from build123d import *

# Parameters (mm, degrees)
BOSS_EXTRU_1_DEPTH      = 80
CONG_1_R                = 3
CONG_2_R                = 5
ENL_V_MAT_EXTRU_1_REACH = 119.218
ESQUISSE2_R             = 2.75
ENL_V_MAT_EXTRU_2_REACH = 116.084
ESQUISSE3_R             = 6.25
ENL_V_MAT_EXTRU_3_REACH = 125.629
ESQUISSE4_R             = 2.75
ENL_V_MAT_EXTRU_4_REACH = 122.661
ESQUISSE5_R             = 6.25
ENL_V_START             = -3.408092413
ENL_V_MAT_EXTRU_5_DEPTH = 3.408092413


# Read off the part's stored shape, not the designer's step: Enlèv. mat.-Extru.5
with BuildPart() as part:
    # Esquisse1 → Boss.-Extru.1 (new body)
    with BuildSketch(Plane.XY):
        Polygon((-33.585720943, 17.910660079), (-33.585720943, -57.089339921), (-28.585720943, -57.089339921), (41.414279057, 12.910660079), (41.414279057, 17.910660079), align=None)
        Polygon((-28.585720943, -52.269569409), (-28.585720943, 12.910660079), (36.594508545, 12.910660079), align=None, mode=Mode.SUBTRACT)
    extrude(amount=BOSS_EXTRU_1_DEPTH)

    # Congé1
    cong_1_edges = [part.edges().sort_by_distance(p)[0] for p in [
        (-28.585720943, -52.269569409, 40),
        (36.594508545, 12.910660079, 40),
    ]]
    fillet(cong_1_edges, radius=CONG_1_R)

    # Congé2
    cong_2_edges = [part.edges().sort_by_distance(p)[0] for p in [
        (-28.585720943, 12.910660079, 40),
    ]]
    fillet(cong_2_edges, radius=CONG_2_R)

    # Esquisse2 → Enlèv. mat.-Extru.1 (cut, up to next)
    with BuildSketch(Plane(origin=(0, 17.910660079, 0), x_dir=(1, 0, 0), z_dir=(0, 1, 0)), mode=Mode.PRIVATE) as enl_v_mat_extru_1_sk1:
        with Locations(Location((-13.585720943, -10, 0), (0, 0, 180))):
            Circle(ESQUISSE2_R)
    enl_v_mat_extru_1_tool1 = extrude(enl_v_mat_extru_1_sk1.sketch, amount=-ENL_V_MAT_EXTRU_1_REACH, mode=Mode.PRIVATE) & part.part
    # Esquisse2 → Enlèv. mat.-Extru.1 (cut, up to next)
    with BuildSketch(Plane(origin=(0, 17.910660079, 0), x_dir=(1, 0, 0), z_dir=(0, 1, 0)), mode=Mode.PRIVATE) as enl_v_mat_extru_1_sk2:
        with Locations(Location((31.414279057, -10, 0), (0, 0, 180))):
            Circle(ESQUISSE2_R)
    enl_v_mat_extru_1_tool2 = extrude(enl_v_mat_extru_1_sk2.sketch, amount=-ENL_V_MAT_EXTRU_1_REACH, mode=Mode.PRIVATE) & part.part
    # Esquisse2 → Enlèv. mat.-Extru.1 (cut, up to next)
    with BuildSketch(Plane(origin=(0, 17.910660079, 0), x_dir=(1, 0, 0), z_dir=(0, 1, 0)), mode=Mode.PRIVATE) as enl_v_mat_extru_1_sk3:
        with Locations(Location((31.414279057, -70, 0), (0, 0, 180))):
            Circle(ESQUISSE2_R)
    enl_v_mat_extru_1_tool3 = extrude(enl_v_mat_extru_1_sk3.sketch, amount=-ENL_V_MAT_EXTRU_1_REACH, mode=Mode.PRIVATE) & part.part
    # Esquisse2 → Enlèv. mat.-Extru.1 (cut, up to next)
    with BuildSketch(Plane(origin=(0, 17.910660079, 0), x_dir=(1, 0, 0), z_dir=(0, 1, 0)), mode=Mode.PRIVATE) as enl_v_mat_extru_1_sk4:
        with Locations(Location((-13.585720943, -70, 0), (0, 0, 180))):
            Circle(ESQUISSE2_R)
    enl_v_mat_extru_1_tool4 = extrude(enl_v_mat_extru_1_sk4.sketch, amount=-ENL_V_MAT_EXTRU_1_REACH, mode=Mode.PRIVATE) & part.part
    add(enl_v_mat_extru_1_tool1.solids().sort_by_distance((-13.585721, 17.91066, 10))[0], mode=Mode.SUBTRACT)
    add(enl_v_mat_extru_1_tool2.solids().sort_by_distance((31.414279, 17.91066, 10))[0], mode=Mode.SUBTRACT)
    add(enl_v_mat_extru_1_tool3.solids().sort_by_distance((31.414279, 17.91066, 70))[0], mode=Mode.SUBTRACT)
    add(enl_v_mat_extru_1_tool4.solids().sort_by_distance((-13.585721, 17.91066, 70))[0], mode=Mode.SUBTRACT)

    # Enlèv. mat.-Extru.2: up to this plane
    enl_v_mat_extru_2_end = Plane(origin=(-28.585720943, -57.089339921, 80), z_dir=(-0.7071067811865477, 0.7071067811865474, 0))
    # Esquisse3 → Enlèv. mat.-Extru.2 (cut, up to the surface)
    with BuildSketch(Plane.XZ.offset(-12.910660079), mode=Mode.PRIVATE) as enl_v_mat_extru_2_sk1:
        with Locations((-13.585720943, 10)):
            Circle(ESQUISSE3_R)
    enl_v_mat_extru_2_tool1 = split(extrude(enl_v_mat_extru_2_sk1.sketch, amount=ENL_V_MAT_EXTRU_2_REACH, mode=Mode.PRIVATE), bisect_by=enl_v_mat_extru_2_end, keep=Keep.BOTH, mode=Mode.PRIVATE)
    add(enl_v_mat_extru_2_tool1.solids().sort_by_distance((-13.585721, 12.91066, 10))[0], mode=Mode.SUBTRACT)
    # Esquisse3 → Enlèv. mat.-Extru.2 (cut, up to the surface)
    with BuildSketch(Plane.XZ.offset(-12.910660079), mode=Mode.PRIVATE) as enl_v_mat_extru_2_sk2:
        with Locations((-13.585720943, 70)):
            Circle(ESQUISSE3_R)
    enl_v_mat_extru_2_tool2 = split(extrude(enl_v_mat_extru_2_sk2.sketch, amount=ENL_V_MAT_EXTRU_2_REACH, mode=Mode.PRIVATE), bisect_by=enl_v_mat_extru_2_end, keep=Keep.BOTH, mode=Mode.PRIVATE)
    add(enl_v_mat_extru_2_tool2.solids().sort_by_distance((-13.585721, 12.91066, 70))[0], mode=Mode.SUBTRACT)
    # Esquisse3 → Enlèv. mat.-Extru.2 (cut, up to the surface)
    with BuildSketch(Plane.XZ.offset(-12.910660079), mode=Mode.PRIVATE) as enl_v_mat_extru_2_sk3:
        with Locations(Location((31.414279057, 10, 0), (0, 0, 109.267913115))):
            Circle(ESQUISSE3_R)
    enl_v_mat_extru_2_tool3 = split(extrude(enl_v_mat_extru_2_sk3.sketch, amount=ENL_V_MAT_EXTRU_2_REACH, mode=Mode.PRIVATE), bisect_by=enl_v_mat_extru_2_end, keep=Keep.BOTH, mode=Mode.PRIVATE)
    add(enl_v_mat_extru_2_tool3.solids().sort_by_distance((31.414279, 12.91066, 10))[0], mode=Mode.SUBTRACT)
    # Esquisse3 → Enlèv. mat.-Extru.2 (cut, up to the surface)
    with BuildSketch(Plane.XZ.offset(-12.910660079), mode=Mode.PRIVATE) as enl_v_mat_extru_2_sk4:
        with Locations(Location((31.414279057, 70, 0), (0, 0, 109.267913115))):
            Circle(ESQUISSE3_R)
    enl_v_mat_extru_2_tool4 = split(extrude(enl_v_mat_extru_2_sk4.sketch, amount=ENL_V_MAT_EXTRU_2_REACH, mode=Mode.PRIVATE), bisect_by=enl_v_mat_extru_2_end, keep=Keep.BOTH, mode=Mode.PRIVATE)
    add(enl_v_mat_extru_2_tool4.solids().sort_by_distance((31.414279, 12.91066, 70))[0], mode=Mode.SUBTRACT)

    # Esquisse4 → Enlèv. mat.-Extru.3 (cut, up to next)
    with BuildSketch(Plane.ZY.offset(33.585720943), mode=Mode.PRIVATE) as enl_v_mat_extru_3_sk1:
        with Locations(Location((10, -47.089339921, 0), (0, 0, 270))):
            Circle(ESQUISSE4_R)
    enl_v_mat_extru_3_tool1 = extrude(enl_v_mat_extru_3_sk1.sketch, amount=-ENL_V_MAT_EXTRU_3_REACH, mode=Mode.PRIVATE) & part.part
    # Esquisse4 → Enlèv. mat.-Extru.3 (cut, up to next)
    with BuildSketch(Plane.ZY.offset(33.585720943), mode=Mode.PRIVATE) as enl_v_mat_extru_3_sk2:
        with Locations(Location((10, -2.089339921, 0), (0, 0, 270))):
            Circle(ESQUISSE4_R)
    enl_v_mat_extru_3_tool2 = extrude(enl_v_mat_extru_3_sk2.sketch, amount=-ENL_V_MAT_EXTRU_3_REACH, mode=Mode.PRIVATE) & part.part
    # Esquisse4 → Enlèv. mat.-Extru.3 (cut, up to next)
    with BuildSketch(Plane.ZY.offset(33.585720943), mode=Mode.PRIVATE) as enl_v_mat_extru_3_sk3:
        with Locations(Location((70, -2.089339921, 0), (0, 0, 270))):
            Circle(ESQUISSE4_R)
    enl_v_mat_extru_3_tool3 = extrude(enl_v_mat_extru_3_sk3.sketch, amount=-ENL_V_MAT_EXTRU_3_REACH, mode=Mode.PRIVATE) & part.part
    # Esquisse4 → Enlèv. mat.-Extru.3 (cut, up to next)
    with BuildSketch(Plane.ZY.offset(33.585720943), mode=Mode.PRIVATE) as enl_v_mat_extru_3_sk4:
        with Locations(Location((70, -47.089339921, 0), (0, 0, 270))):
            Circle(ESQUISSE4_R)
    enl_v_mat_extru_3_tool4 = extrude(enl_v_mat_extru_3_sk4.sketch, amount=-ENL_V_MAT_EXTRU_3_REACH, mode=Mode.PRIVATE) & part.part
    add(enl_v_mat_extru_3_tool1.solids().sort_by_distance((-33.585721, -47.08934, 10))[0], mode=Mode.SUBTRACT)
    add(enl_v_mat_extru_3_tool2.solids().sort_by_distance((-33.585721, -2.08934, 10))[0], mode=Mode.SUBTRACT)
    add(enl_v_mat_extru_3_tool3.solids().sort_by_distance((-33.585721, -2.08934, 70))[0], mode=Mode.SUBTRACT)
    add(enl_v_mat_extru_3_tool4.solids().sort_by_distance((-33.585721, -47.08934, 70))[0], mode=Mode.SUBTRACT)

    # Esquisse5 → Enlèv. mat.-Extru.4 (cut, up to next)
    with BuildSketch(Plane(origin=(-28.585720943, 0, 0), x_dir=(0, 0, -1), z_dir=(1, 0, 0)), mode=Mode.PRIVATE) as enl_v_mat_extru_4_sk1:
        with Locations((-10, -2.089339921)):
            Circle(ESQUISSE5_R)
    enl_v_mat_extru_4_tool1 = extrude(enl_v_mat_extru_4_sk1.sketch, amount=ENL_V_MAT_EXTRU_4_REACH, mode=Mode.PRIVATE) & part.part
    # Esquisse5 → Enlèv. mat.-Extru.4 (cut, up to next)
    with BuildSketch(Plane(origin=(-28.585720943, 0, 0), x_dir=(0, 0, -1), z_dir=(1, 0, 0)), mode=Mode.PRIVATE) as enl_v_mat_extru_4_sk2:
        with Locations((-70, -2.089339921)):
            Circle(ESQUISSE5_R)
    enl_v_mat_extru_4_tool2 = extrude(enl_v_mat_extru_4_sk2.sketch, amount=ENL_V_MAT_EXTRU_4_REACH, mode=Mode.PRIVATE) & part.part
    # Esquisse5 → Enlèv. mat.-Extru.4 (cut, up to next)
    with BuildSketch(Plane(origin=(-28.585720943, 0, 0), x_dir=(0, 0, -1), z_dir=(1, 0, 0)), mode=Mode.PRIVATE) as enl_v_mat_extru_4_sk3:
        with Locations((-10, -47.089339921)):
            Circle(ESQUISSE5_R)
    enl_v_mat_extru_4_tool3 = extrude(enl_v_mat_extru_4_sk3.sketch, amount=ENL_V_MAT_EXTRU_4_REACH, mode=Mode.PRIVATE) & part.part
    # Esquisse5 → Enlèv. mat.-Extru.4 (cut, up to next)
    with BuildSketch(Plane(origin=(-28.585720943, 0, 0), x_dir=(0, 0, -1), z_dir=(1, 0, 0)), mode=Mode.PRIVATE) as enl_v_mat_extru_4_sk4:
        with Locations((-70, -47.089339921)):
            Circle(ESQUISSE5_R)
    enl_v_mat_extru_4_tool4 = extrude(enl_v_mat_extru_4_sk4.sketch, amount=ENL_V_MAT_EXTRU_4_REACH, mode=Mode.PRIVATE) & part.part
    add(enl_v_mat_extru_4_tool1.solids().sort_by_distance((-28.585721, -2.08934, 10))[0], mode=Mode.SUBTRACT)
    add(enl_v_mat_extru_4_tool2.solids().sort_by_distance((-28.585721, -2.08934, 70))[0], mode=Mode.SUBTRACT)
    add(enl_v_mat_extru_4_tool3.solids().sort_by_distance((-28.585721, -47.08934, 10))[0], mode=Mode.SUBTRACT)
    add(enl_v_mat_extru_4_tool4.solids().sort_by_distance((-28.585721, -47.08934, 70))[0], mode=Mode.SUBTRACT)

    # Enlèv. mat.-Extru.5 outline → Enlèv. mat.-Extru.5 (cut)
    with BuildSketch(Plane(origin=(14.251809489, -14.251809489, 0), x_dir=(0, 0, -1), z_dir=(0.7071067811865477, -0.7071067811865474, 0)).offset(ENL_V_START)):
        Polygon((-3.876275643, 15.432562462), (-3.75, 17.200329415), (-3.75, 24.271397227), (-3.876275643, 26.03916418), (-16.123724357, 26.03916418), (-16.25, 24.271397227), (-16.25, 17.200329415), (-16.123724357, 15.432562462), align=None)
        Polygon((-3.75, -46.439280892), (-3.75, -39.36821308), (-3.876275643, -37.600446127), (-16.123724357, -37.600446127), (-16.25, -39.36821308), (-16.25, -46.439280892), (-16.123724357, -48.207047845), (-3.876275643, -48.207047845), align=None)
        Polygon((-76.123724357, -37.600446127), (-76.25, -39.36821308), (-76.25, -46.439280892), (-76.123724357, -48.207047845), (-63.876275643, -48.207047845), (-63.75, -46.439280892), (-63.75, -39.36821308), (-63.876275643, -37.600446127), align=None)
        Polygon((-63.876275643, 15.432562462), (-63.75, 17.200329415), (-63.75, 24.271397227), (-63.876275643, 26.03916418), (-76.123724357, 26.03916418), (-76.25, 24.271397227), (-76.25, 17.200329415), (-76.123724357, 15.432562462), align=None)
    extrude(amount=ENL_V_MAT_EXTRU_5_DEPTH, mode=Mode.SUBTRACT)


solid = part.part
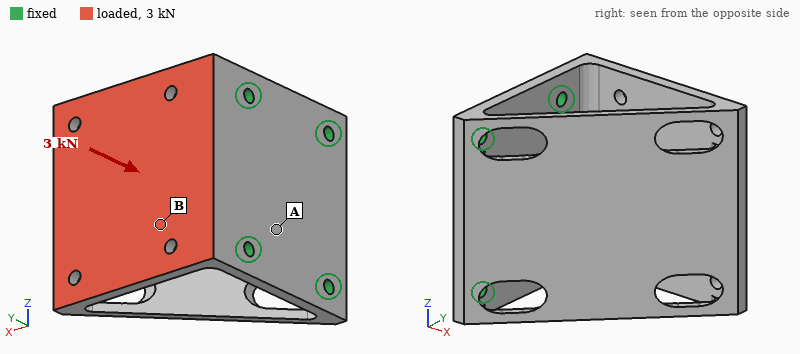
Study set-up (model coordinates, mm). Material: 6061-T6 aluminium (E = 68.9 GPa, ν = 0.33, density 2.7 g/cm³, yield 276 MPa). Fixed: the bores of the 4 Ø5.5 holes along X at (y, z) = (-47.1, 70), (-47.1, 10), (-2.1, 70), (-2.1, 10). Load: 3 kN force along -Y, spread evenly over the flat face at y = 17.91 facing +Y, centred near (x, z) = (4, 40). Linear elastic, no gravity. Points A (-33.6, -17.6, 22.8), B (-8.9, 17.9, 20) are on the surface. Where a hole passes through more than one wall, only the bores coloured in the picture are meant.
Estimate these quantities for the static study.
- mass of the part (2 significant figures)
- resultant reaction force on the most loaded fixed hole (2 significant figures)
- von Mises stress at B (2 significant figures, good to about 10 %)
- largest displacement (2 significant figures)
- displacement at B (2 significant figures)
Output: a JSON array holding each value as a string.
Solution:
["220 g", "1.1 kN", "30 MPa", "0.25 mm", "0.18 mm"]
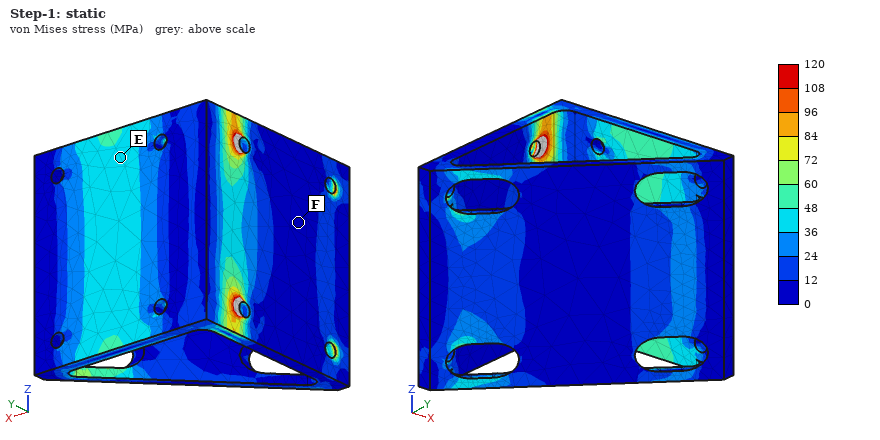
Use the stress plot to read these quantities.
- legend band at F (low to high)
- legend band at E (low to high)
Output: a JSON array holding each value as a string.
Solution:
["0 to 12 MPa", "36 to 48 MPa"]
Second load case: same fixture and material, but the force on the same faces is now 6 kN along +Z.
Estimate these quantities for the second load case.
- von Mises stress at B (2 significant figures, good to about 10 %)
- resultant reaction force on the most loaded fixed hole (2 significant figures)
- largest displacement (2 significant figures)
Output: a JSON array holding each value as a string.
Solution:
["23 MPa", "3.2 kN", "0.20 mm"]
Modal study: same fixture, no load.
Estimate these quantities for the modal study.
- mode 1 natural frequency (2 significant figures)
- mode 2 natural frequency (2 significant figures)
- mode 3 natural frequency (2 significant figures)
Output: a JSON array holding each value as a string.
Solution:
["1500 Hz", "2400 Hz", "2500 Hz"]
